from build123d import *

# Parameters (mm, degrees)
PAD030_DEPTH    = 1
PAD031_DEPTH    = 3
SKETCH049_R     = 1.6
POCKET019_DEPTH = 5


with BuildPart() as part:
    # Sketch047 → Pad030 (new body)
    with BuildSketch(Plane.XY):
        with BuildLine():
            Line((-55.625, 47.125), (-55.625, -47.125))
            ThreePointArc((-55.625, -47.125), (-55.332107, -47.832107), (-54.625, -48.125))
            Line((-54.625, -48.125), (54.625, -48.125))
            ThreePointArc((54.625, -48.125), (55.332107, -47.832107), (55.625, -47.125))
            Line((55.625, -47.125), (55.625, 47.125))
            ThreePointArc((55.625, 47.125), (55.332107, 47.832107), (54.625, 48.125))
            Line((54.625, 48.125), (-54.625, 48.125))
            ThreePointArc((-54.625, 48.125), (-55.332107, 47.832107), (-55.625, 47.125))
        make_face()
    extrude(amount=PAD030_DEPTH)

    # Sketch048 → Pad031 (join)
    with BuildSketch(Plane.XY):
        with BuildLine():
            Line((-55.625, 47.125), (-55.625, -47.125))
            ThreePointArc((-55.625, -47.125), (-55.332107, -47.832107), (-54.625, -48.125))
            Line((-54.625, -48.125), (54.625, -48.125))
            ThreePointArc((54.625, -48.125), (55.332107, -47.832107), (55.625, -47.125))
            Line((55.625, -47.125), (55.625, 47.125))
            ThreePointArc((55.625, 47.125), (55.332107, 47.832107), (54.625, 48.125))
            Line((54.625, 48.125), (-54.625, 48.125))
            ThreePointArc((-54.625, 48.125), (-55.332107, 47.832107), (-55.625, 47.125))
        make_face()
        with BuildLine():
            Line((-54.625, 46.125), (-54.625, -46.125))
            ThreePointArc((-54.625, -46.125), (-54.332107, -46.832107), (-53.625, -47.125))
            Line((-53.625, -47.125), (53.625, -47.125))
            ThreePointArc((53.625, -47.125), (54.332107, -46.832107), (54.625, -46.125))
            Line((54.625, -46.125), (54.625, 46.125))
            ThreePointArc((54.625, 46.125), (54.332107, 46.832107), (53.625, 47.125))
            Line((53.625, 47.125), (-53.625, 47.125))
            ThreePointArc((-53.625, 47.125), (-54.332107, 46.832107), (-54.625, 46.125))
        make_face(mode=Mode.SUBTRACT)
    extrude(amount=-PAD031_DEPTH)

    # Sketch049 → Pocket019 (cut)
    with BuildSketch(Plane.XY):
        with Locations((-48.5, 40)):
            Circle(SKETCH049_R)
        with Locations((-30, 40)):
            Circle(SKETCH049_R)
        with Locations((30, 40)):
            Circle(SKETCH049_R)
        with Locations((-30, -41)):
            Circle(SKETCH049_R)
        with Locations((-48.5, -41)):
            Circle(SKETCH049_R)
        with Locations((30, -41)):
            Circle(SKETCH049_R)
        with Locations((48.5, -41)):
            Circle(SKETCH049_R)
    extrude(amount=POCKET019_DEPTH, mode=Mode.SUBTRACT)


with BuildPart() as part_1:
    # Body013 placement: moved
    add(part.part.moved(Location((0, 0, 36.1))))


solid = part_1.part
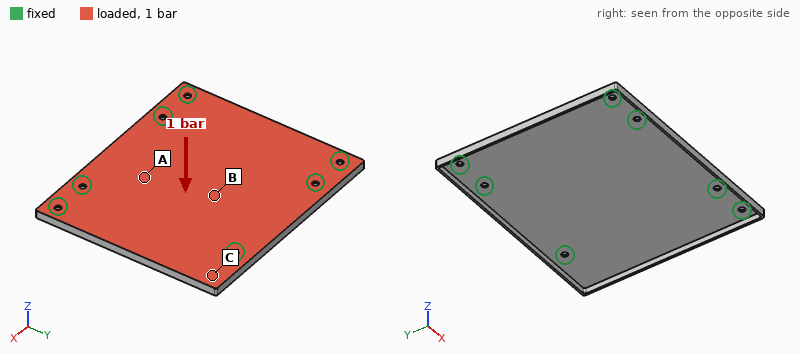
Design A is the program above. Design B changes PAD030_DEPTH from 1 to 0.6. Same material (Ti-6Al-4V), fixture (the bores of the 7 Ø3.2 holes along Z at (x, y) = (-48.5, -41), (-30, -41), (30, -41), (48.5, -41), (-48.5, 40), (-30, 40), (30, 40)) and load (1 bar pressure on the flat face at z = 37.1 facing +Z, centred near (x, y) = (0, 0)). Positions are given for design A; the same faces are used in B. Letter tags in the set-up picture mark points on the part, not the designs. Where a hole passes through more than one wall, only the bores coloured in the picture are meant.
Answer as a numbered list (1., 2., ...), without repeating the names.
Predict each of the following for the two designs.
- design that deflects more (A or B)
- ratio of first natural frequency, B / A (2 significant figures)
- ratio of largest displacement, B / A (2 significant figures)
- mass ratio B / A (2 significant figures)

1. B
2. 0.63
3. 4.3
4. 0.64
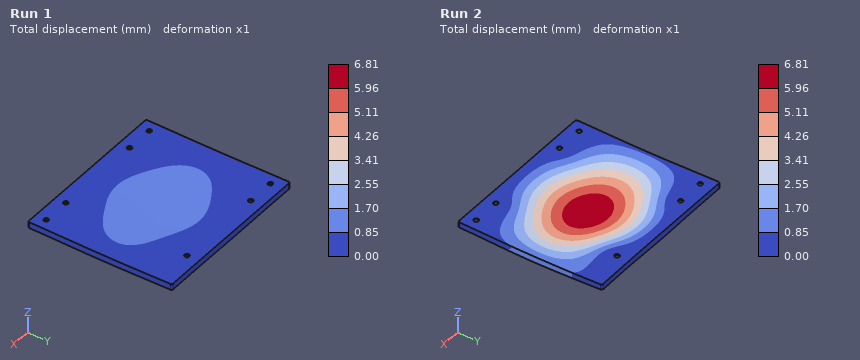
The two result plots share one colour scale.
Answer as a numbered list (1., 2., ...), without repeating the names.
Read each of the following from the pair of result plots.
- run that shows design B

1. Run 2
